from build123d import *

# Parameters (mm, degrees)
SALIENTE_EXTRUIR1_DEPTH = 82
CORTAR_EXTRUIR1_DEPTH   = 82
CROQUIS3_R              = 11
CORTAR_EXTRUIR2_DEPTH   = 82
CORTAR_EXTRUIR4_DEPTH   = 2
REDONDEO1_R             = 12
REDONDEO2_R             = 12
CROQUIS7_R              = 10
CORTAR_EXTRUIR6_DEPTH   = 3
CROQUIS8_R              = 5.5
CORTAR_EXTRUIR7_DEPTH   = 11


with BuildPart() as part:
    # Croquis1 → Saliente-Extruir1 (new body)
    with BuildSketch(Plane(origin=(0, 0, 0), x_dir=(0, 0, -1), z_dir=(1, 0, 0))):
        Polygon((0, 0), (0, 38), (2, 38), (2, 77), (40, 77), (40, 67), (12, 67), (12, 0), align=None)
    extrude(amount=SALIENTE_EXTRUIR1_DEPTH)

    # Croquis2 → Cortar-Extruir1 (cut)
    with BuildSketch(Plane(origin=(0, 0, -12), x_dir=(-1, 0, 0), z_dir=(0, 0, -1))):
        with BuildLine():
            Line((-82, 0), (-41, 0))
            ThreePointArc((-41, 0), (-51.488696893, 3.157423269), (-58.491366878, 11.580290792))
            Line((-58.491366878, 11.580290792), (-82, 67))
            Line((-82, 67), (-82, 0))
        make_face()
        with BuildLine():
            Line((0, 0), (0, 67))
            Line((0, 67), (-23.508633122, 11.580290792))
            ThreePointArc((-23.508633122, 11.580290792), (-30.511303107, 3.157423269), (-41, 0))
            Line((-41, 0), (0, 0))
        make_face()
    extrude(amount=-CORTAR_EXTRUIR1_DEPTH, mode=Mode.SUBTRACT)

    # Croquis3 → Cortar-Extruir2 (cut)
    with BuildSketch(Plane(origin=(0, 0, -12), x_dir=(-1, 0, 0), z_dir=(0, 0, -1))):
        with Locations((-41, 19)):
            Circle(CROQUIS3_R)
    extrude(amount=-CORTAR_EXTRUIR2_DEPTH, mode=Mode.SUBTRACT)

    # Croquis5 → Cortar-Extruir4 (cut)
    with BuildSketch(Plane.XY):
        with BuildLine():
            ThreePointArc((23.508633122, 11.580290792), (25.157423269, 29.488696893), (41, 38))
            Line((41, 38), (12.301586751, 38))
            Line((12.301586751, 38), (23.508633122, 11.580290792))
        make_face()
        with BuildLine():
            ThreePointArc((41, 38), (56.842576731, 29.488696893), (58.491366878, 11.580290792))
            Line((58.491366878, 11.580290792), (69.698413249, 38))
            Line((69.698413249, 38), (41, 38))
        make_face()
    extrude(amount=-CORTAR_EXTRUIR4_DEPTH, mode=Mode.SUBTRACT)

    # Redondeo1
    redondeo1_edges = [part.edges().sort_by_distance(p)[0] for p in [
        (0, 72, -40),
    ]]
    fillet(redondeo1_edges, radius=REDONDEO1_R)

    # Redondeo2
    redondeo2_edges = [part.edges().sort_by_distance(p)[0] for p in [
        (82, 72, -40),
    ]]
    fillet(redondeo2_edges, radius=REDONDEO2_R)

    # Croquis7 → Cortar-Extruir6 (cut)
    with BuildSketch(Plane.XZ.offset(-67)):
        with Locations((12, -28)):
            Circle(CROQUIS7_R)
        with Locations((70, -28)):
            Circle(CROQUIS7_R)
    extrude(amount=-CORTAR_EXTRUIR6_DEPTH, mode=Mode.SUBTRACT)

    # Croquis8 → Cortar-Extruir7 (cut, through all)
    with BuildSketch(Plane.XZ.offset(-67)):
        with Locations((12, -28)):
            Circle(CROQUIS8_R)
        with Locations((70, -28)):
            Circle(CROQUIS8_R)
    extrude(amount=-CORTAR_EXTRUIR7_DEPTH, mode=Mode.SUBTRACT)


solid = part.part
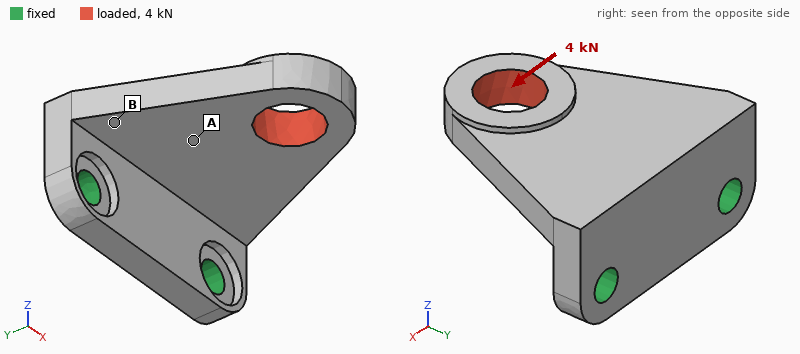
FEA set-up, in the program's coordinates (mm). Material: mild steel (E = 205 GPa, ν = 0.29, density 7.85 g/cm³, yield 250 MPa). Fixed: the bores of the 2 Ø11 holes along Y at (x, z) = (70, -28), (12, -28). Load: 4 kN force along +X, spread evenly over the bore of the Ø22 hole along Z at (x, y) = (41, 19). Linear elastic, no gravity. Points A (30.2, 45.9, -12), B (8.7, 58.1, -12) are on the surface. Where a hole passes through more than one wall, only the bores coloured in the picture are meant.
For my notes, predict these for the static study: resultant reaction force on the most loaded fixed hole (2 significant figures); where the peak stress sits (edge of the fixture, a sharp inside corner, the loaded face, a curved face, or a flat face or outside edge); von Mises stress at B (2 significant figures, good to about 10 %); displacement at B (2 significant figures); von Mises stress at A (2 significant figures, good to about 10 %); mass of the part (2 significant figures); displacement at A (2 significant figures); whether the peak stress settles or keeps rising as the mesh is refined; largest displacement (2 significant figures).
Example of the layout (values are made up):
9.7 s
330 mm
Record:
4.3 kN
edge of the fixture
46 MPa
19 µm
20 MPa
470 g
18 µm
keeps rising
50 µm
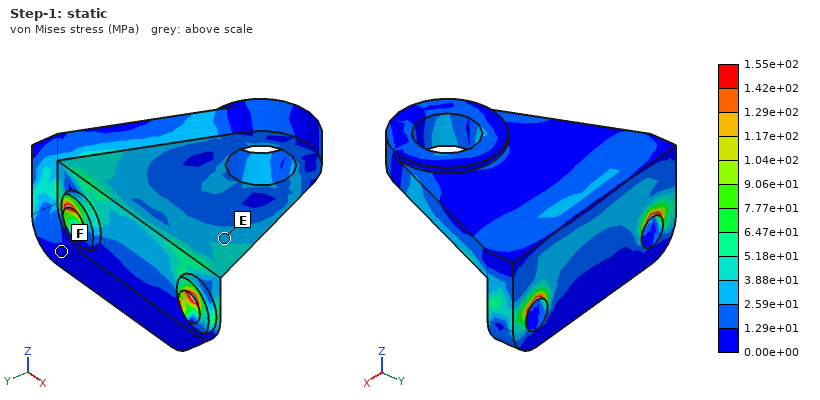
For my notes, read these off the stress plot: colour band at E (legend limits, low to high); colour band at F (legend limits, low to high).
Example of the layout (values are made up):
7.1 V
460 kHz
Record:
2.59e+01 to 3.88e+01 MPa
0.00e+00 to 1.29e+01 MPa
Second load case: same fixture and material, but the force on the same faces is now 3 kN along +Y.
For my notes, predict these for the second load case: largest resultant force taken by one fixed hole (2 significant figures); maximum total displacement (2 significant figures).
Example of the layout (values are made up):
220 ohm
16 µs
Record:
1.5 kN
68 µm
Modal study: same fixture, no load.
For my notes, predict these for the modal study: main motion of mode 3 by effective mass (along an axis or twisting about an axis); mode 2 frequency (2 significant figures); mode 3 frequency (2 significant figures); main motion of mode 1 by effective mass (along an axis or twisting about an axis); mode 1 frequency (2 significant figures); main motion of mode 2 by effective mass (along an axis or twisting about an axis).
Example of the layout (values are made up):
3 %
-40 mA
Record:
along Y
4300 Hz
5500 Hz
along Z
1500 Hz
along X
